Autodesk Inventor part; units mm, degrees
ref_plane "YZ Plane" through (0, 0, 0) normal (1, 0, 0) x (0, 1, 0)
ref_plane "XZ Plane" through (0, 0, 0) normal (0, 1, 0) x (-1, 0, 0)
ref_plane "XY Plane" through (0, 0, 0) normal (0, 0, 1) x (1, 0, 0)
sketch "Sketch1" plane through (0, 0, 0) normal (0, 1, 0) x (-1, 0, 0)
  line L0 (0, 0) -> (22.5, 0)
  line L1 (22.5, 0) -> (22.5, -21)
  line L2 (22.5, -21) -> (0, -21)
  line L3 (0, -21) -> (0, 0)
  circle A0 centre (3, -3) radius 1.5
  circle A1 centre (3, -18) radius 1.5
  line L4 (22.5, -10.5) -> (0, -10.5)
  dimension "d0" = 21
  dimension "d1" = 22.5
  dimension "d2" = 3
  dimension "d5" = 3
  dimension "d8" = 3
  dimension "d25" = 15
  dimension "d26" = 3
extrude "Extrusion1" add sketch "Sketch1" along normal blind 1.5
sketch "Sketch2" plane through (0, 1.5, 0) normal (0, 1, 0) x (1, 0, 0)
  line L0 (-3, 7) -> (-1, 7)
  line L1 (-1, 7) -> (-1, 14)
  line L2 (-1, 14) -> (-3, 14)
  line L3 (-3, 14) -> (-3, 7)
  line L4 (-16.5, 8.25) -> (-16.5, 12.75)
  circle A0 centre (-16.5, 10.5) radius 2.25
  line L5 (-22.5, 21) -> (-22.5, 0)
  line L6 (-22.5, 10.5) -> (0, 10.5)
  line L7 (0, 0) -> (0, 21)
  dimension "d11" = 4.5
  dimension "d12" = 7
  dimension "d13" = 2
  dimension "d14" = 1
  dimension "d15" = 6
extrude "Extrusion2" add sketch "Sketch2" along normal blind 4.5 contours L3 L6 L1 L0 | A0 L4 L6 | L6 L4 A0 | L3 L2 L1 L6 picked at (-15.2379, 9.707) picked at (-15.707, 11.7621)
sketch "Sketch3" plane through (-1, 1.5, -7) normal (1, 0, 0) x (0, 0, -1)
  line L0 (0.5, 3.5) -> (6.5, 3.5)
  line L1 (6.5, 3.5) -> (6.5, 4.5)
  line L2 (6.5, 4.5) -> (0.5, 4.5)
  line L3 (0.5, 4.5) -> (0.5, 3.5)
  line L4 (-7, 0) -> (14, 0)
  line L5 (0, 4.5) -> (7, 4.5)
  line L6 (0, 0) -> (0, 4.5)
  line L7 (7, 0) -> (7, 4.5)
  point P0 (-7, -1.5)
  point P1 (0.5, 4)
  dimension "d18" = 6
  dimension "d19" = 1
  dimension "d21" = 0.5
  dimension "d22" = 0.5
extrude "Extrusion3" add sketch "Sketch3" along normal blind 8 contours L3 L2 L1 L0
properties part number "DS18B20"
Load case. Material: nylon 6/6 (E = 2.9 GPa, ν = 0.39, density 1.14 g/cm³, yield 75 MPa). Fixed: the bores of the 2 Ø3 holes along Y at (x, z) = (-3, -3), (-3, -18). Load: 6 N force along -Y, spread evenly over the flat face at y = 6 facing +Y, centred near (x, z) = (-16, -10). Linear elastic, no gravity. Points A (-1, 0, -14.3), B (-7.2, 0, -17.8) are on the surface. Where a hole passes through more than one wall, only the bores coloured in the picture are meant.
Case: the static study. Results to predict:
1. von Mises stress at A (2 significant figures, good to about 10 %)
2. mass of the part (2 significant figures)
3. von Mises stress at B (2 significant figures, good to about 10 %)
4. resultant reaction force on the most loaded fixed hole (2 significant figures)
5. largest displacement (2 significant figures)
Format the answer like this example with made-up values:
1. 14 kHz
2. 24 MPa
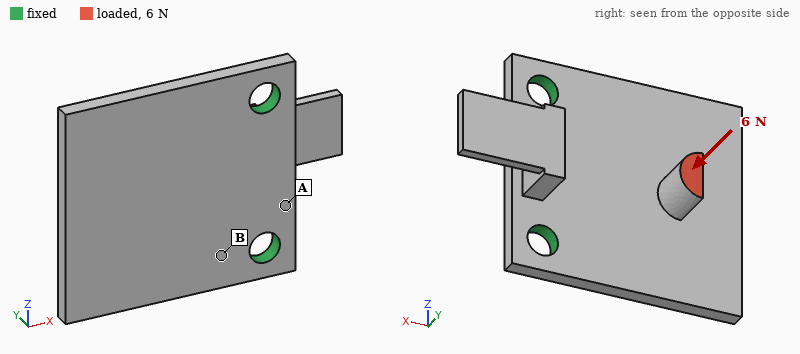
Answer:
1. 2.3 MPa
2. 0.95 g
3. 6.6 MPa
4. 3.0 N
5. 0.39 mm
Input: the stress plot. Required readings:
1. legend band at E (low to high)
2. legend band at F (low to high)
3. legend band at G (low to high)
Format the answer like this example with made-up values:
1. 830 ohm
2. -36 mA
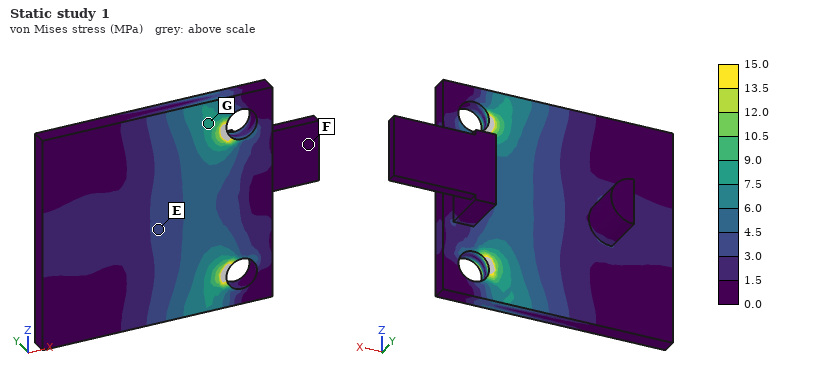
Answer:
1. 3.0 to 4.5 MPa
2. 0.0 to 1.5 MPa
3. 7.5 to 9.0 MPa
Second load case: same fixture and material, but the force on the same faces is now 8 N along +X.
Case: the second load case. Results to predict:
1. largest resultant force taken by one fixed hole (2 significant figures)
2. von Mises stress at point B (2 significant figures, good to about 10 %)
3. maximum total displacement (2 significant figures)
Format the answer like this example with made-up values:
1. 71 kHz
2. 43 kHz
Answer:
1. 4.3 N
2. 4.9 MPa
3. 0.37 mm
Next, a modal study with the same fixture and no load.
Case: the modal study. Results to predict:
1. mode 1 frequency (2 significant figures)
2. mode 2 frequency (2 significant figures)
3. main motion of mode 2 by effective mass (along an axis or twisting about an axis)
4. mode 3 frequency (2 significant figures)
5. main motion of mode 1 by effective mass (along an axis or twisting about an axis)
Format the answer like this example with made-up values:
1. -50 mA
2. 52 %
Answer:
1. 1100 Hz
2. 2500 Hz
3. twisting about X
4. 3000 Hz
5. along Y
